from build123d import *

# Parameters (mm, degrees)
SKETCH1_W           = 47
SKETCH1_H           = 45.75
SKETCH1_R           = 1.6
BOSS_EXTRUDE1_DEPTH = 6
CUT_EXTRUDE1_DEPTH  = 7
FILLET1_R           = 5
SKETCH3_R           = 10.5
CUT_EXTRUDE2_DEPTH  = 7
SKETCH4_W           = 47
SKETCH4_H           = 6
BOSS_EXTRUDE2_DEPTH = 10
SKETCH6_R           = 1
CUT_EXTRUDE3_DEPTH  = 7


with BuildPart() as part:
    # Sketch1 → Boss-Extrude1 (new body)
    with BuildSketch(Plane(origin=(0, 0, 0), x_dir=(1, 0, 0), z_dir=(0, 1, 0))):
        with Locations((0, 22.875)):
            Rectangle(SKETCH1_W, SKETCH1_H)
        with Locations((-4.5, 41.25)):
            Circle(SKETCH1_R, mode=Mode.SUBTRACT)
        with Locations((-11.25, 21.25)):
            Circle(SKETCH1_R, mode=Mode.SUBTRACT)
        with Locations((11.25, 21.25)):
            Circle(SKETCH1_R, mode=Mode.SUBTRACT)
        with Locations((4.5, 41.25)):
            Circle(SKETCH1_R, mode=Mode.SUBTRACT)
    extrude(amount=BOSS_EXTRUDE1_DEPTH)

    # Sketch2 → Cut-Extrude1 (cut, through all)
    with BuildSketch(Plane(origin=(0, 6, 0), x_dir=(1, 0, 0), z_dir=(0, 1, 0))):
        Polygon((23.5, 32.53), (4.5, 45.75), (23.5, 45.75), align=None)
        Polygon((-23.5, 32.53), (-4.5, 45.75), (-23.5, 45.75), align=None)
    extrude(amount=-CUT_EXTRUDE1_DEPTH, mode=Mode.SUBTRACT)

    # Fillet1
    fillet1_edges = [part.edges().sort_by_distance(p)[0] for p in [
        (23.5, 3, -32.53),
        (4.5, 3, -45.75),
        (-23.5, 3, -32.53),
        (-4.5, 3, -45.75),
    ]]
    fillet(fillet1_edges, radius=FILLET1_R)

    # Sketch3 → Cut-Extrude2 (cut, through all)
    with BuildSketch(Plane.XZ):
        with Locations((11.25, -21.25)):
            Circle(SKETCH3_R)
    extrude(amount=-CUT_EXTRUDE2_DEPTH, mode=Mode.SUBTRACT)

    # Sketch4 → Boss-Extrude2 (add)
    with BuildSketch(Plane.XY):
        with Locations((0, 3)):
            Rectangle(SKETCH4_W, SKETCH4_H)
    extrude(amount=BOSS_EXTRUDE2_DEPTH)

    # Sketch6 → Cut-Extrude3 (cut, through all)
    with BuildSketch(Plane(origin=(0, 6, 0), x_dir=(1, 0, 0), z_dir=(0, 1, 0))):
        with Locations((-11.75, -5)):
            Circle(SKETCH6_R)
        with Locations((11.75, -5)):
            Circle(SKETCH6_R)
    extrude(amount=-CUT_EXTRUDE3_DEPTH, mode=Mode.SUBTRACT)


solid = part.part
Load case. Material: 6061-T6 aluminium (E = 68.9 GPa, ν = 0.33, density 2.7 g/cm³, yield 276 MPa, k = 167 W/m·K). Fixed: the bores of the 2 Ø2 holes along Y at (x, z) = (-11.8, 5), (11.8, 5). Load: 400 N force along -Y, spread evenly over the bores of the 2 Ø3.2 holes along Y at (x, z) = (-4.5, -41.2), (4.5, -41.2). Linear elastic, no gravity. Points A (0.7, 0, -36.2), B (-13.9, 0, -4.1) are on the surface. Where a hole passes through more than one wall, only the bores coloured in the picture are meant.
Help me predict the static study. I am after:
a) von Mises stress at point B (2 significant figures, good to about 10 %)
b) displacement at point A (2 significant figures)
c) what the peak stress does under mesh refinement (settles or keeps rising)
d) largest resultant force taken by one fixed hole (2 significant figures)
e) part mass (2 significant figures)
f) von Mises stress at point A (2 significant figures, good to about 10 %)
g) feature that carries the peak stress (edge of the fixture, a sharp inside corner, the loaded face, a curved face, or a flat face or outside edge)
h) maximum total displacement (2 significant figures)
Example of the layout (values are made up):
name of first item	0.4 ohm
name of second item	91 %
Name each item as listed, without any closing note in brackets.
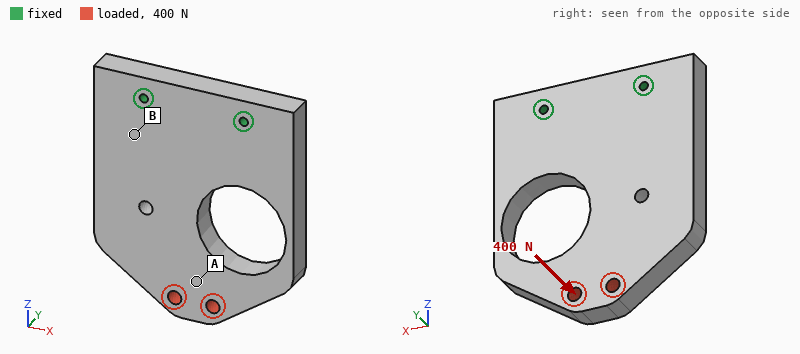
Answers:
von Mises stress at point B	61 MPa
displacement at point A	0.32 mm
what the peak stress does under mesh refinement	keeps rising
largest resultant force taken by one fixed hole	210 N
part mass	32 g
von Mises stress at point A	26 MPa
feature that carries the peak stress	edge of the fixture
maximum total displacement	0.44 mm
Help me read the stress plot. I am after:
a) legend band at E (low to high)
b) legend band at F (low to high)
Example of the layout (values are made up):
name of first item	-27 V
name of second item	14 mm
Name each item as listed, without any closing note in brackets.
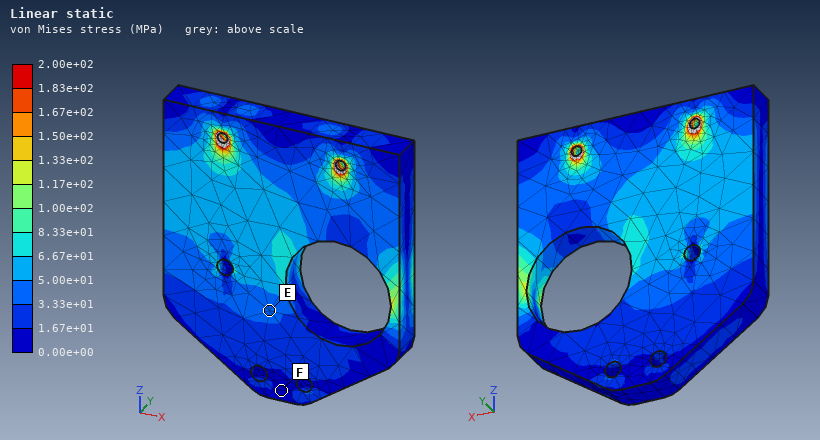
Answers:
legend band at E	3.33e+01 to 5.00e+01 MPa
legend band at F	0.00e+00 to 1.67e+01 MPa
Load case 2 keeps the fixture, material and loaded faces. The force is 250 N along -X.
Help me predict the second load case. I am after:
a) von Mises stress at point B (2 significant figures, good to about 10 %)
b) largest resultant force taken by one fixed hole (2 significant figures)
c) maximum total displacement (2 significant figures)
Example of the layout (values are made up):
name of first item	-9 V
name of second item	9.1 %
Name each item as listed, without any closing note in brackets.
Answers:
von Mises stress at point B	5.0 MPa
largest resultant force taken by one fixed hole	500 N
maximum total displacement	14 µm
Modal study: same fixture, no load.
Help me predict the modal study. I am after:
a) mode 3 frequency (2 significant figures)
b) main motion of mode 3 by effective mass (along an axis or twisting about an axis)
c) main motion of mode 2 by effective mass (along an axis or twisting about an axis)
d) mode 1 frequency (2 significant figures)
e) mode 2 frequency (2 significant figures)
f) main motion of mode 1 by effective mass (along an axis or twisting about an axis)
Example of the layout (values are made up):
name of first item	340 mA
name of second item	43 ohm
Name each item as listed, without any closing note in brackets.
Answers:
mode 3 frequency	7400 Hz
main motion of mode 3 by effective mass	along X
main motion of mode 2 by effective mass	twisting about Z
mode 1 frequency	2000 Hz
mode 2 frequency	5300 Hz
main motion of mode 1 by effective mass	along Y
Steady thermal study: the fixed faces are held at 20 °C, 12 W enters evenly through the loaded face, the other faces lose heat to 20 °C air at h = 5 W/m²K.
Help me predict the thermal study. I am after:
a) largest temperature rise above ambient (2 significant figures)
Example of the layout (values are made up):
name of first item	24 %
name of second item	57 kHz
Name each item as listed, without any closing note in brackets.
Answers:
largest temperature rise above ambient	23 K
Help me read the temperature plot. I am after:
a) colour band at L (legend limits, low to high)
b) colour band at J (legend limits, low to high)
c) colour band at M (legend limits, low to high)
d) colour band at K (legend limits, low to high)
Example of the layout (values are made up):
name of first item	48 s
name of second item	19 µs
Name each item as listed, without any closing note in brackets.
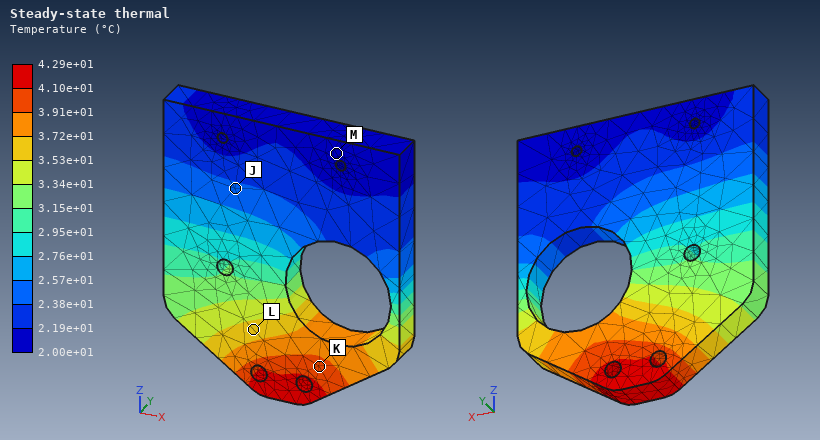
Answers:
colour band at L	3.53e+01 to 3.72e+01 °C
colour band at J	2.38e+01 to 2.57e+01 °C
colour band at M	2.00e+01 to 2.19e+01 °C
colour band at K	3.91e+01 to 4.10e+01 °C
